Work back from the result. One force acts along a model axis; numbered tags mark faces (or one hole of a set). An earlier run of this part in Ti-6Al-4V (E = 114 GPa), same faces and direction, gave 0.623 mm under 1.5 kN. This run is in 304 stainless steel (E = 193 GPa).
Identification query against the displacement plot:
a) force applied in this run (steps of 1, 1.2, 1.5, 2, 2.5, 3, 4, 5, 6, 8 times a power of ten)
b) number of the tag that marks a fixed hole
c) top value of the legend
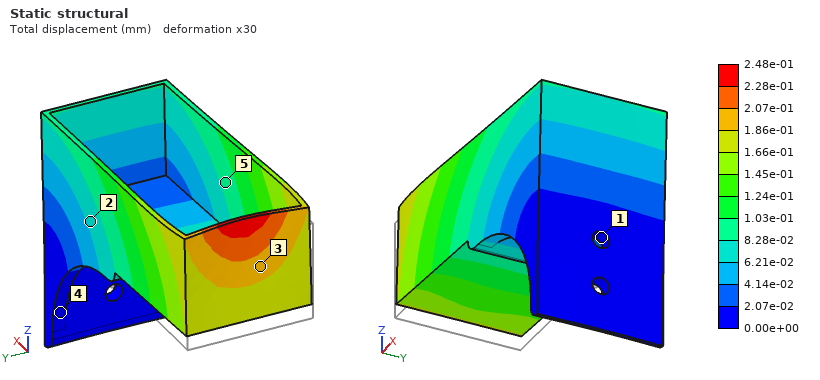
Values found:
1 kN
1
2.48e-01 mm
